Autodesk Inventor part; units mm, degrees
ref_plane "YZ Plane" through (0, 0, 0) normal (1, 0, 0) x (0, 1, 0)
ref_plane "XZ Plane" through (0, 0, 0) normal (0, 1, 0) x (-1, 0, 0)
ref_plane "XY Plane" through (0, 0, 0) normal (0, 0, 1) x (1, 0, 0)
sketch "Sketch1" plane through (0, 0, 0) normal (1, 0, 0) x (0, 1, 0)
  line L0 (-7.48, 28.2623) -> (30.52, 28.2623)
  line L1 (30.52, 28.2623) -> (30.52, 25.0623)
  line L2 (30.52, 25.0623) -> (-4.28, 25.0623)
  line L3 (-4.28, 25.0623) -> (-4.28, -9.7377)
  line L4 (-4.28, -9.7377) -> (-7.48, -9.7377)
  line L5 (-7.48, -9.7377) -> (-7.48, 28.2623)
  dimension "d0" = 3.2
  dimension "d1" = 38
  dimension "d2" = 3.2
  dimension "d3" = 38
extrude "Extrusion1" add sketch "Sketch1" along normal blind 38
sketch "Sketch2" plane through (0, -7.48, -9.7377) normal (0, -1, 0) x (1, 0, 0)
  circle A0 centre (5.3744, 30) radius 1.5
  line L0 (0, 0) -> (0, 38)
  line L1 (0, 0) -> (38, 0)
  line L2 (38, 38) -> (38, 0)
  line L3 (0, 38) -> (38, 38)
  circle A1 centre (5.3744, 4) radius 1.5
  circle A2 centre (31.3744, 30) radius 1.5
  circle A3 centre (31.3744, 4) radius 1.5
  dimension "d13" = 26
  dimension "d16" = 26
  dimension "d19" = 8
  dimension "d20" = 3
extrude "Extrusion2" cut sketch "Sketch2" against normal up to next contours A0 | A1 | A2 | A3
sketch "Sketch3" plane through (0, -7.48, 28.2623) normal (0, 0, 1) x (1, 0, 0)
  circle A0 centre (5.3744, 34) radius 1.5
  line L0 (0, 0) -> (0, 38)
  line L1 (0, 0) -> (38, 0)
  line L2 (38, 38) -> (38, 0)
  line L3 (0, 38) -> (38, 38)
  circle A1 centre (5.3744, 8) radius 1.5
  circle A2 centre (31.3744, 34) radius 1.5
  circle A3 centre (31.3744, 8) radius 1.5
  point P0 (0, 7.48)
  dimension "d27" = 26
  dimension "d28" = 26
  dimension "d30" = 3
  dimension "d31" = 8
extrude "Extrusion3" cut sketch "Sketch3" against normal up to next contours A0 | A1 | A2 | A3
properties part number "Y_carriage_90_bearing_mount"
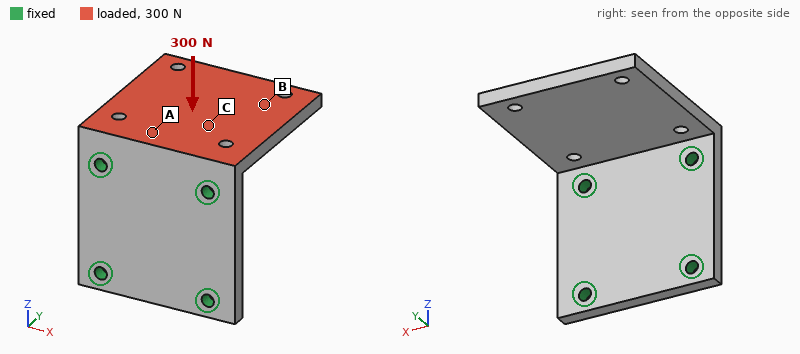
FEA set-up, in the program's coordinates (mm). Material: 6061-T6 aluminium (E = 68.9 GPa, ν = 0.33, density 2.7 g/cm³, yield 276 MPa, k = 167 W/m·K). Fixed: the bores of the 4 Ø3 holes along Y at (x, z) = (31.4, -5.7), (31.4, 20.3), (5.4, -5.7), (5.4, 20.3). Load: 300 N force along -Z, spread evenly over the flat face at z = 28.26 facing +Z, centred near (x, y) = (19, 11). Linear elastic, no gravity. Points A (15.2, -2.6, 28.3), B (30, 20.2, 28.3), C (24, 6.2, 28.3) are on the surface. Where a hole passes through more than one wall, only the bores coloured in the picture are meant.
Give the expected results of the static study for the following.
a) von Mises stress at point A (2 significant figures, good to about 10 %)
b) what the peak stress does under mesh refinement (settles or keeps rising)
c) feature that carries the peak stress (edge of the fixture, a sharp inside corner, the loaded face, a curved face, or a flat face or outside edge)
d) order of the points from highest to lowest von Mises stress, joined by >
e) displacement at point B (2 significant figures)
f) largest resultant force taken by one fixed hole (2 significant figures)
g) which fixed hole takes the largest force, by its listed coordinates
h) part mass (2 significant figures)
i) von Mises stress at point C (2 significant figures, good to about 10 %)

63 MPa
keeps rising
edge of the fixture
A > C > B
0.26 mm
130 N
(31.4, 20.3)
23 g
32 MPa
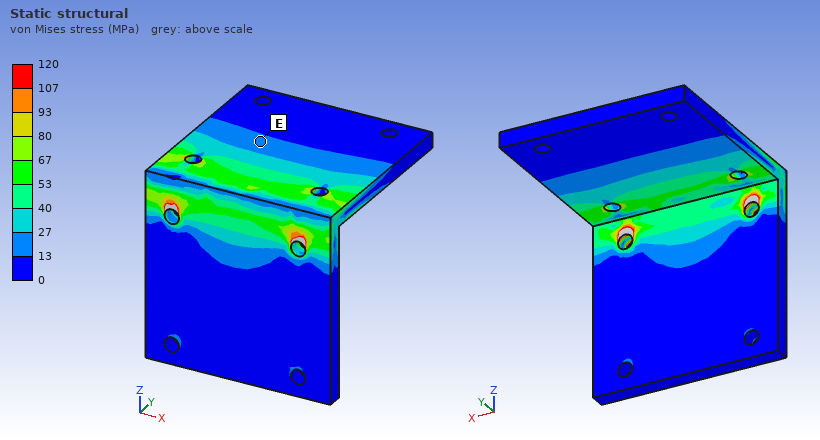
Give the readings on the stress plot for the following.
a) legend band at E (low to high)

13 to 27 MPa
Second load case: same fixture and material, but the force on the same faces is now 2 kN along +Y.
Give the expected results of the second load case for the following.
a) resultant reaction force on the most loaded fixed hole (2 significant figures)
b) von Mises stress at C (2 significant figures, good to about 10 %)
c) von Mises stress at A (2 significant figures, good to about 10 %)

1.1 kN
38 MPa
56 MPa
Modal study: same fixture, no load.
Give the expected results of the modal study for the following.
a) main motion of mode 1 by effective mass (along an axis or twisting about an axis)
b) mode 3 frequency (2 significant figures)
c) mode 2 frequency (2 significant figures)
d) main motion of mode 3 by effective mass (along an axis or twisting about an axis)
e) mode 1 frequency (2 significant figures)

along Z
6900 Hz
4100 Hz
along X
1600 Hz
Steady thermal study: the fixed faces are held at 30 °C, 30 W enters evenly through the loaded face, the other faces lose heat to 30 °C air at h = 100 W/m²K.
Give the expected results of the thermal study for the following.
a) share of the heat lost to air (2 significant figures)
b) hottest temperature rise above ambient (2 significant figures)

17 %
31 K
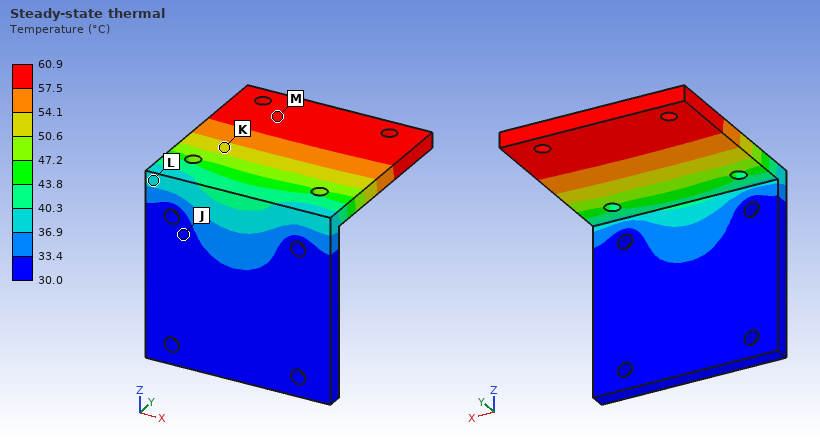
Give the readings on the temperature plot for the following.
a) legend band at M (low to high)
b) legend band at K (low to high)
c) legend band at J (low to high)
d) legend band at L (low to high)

57.5 to 60.9 °C
50.6 to 54.1 °C
30.0 to 33.4 °C
36.9 to 40.3 °C
